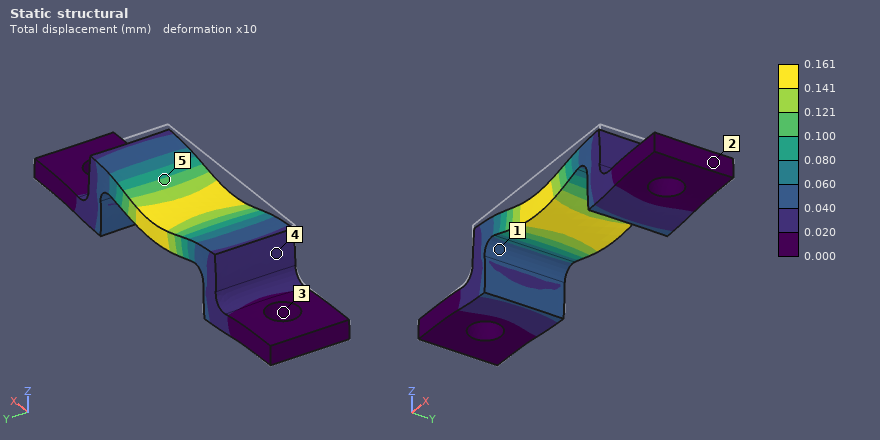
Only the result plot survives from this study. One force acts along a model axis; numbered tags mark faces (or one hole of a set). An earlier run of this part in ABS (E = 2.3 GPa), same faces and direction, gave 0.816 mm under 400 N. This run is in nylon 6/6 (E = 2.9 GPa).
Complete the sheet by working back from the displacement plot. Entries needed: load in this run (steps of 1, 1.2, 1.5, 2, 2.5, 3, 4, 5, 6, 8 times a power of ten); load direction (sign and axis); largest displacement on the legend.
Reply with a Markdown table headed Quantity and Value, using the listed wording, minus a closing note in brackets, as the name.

| Quantity | Value |
|---|---|
| load in this run | 100 N |
| load direction | -Z |
| largest displacement on the legend | 0.161 mm |
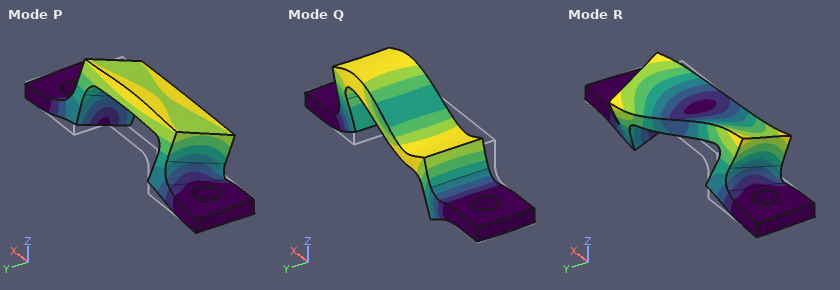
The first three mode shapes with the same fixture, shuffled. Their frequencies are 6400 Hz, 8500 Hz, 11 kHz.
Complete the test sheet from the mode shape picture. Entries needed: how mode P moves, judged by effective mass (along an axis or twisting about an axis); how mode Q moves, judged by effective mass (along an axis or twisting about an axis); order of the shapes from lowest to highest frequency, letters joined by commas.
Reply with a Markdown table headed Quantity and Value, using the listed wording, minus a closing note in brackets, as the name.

| Quantity | Value |
|---|---|
| how mode P moves, judged by effective mass | along Y |
| how mode Q moves, judged by effective mass | along X |
| order of the shapes from lowest to highest frequency, letters joined by commas | P, Q, R |
